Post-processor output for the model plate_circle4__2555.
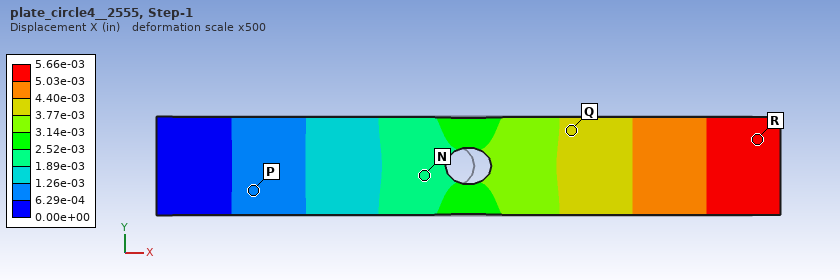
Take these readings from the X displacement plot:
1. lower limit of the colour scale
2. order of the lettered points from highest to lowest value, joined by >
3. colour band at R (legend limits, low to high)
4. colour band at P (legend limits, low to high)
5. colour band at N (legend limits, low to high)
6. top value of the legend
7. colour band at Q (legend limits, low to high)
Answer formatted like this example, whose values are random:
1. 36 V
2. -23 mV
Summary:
1. 0.00e+00 in
2. R > Q > N > P
3. 5.03e-03 to 5.66e-03 in
4. 6.29e-04 to 1.26e-03 in
5. 1.89e-03 to 2.52e-03 in
6. 5.66e-03 in
7. 3.77e-03 to 4.40e-03 in
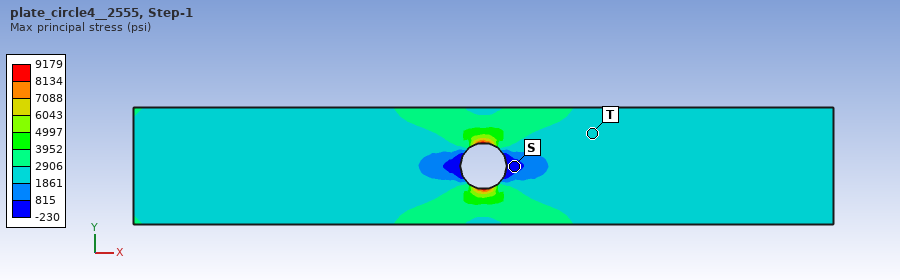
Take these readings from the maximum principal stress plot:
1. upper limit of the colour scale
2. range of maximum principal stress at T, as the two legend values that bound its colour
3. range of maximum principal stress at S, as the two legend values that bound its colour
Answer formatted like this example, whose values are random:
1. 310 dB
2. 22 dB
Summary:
1. 9179 psi
2. 1861 to 2906 psi
3. -230 to 815 psi
